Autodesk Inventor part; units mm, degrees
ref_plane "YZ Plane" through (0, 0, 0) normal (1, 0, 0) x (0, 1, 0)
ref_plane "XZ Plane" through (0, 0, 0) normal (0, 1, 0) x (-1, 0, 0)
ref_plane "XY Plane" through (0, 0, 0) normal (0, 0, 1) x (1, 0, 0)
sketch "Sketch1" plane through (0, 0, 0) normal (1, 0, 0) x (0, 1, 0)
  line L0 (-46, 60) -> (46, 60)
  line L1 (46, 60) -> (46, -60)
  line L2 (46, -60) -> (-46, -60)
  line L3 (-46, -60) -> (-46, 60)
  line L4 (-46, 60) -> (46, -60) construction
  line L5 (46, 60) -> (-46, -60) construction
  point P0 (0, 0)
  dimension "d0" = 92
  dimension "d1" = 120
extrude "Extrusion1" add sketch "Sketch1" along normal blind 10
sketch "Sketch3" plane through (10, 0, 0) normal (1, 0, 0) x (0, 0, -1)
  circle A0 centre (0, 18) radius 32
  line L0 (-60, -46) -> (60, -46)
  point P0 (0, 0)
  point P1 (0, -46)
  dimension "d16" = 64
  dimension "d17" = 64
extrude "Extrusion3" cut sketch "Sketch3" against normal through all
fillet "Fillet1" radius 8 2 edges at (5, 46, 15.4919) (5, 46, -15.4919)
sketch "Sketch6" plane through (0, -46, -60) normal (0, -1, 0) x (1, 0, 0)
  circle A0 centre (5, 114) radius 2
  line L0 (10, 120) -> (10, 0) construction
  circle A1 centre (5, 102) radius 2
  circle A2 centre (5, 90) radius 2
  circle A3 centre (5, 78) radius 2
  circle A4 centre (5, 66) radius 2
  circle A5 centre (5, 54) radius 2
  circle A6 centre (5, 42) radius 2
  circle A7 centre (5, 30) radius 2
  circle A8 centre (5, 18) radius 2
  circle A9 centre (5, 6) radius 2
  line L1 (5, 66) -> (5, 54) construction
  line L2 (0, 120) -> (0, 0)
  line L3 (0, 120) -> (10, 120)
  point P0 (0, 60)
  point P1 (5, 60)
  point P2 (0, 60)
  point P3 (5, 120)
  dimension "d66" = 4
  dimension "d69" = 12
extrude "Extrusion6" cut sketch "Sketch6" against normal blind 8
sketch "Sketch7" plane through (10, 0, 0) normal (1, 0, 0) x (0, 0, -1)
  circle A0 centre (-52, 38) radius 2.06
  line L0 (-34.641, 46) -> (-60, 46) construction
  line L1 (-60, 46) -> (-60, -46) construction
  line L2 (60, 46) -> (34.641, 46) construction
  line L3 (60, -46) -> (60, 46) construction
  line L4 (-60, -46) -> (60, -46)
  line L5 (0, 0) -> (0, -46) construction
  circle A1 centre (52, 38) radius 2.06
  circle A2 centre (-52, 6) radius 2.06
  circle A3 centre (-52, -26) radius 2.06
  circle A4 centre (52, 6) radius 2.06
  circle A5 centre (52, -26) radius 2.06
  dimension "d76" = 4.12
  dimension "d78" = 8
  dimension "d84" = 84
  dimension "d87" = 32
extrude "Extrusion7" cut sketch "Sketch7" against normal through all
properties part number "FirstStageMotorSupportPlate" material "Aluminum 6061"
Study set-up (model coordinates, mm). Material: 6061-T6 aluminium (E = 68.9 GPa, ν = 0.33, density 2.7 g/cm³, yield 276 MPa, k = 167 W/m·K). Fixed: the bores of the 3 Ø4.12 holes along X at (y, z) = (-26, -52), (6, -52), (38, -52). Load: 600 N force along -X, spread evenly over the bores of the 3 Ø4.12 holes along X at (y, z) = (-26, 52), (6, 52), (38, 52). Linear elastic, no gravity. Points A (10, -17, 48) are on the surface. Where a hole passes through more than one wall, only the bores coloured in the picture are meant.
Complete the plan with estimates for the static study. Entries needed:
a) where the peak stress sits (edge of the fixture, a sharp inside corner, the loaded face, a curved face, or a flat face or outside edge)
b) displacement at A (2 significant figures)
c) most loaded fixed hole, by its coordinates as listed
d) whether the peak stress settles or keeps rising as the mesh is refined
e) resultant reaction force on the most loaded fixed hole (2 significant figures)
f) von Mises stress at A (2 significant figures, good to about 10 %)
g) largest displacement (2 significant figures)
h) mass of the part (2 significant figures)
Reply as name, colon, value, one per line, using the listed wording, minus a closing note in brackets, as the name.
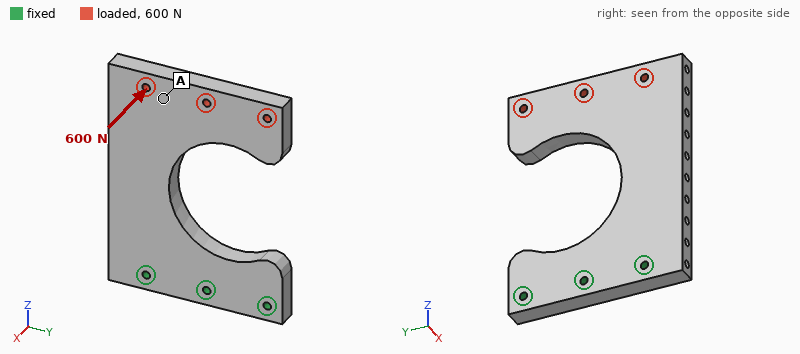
where the peak stress sits: edge of the fixture
displacement at A: 0.99 mm
most loaded fixed hole, by its coordinates as listed: (6, -52)
whether the peak stress settles or keeps rising as the mesh is refined: keeps rising
resultant reaction force on the most loaded fixed hole: 680 N
von Mises stress at A: 17 MPa
largest displacement: 1.6 mm
mass of the part: 210 g
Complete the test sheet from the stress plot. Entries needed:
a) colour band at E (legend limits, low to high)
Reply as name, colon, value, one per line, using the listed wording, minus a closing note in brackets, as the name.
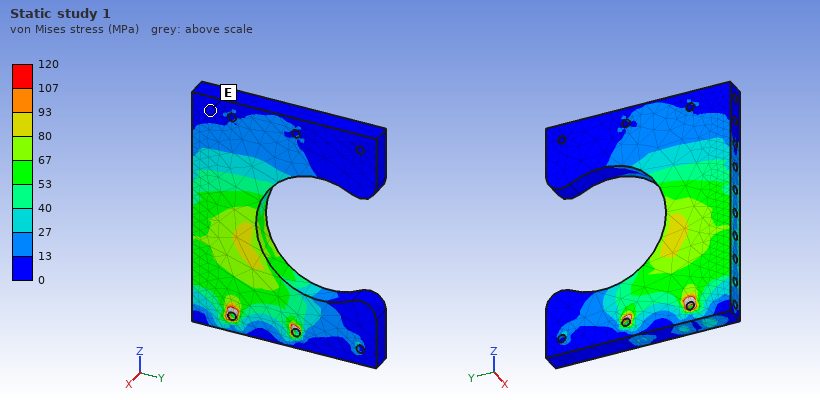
colour band at E: 0 to 13 MPa
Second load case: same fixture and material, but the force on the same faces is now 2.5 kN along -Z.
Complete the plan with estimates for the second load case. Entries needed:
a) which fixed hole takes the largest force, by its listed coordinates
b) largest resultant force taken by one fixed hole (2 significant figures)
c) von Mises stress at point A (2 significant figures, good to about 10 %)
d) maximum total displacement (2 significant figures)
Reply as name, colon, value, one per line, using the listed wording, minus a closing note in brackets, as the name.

which fixed hole takes the largest force, by its listed coordinates: (6, -52)
largest resultant force taken by one fixed hole: 2.1 kN
von Mises stress at point A: 13 MPa
maximum total displacement: 0.32 mm
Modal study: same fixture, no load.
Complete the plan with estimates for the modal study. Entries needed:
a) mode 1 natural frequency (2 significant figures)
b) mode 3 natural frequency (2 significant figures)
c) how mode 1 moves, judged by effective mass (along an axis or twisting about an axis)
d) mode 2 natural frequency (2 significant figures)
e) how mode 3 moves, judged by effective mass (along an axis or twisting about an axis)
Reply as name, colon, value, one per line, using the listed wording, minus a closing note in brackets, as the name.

mode 1 natural frequency: 440 Hz
mode 3 natural frequency: 1400 Hz
how mode 1 moves, judged by effective mass: along X
mode 2 natural frequency: 1100 Hz
how mode 3 moves, judged by effective mass: along Y
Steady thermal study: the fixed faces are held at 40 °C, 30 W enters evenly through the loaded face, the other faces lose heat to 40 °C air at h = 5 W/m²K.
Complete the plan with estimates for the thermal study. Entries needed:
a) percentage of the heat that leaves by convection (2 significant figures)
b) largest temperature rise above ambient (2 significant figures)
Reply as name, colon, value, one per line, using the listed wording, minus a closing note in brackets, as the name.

percentage of the heat that leaves by convection: 8.9 %
largest temperature rise above ambient: 58 K
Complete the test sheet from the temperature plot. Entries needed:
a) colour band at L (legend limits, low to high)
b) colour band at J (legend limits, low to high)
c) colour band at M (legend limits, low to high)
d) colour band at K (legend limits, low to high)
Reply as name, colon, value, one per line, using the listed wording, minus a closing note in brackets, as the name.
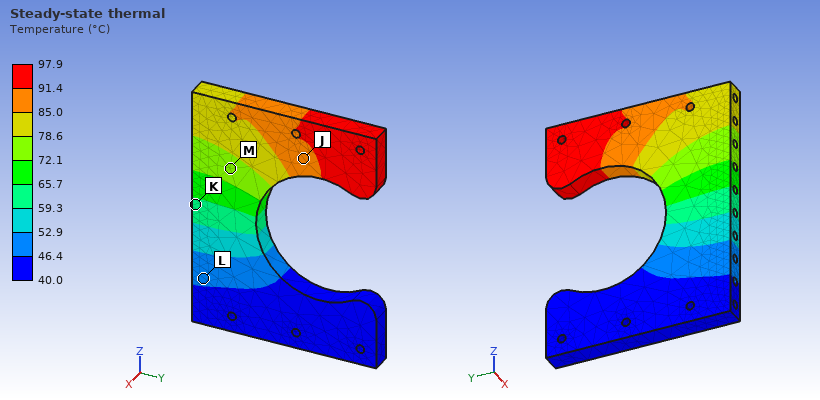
colour band at L: 46.4 to 52.9 °C
colour band at J: 85.0 to 91.4 °C
colour band at M: 72.1 to 78.6 °C
colour band at K: 59.3 to 65.7 °C
